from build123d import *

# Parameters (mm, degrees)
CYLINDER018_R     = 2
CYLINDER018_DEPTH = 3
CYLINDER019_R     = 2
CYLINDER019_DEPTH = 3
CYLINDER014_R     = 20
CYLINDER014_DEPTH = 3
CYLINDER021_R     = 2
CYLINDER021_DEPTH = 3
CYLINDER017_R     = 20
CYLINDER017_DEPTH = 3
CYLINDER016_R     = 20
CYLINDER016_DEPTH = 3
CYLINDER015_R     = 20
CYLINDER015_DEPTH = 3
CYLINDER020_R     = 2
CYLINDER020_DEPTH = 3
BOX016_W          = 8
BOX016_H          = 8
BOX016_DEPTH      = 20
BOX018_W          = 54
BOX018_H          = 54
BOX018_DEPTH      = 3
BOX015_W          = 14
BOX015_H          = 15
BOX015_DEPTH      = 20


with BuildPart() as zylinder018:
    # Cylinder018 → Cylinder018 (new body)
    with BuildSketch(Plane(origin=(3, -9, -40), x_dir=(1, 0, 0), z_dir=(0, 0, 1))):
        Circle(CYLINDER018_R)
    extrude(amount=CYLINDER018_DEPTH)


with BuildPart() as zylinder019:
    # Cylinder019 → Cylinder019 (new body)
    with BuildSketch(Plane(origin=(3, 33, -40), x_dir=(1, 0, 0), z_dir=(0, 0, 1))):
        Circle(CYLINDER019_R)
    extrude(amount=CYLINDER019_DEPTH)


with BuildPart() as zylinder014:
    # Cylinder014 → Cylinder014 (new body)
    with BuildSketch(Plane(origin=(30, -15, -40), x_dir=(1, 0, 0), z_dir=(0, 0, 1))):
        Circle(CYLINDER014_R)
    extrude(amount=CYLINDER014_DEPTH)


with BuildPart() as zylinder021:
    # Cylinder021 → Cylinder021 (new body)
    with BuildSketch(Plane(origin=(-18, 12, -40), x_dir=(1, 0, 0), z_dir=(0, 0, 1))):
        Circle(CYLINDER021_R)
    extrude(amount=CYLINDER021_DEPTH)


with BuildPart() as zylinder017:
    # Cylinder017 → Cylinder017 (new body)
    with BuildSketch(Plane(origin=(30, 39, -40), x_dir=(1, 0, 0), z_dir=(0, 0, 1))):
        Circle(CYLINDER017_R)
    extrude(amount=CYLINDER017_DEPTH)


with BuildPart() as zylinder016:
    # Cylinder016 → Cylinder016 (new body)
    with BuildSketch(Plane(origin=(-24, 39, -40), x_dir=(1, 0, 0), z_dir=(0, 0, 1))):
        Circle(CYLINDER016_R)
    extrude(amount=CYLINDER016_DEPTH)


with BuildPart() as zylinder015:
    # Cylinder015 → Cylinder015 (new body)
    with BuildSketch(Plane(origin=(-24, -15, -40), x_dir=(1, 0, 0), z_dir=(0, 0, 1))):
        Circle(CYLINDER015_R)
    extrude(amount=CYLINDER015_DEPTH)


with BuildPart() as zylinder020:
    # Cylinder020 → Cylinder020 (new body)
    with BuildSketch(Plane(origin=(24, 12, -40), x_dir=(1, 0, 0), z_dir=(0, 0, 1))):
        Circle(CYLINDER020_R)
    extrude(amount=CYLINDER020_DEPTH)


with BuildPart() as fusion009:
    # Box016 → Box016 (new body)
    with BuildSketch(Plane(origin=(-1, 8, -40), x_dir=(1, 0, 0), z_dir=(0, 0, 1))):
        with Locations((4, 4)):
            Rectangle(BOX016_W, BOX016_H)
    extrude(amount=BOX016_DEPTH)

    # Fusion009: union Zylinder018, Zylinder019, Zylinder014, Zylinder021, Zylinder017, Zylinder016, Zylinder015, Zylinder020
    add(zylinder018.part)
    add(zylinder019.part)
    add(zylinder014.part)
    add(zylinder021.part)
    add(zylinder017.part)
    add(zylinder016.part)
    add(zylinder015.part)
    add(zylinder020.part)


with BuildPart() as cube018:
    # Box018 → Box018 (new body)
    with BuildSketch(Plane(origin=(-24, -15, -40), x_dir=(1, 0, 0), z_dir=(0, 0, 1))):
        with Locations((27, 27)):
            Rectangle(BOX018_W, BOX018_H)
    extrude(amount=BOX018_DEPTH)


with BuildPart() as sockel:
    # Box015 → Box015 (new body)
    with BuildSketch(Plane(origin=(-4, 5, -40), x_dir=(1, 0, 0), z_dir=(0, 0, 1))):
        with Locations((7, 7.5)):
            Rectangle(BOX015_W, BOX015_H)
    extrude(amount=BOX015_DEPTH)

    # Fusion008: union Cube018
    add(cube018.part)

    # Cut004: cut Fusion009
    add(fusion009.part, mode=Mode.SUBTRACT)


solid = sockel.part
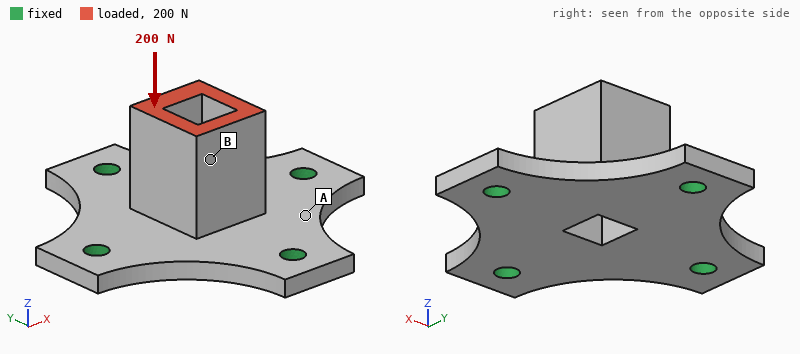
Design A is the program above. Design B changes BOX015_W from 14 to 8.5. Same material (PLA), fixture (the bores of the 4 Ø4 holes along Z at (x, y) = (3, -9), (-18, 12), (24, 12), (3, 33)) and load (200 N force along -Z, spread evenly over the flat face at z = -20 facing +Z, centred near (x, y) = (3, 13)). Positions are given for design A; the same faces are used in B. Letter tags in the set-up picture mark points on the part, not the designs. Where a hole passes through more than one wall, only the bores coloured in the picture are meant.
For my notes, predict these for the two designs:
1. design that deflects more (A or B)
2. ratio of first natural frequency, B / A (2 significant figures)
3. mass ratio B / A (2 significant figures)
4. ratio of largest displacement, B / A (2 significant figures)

B
1.0
0.80
1.5
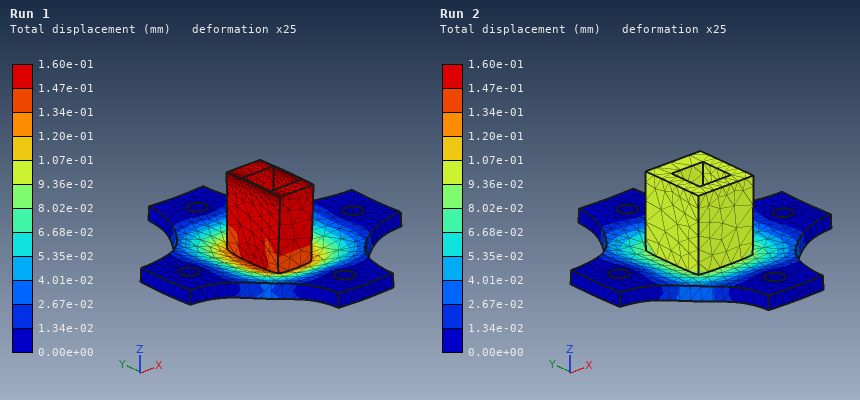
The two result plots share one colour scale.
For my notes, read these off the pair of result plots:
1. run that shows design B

Run 1
